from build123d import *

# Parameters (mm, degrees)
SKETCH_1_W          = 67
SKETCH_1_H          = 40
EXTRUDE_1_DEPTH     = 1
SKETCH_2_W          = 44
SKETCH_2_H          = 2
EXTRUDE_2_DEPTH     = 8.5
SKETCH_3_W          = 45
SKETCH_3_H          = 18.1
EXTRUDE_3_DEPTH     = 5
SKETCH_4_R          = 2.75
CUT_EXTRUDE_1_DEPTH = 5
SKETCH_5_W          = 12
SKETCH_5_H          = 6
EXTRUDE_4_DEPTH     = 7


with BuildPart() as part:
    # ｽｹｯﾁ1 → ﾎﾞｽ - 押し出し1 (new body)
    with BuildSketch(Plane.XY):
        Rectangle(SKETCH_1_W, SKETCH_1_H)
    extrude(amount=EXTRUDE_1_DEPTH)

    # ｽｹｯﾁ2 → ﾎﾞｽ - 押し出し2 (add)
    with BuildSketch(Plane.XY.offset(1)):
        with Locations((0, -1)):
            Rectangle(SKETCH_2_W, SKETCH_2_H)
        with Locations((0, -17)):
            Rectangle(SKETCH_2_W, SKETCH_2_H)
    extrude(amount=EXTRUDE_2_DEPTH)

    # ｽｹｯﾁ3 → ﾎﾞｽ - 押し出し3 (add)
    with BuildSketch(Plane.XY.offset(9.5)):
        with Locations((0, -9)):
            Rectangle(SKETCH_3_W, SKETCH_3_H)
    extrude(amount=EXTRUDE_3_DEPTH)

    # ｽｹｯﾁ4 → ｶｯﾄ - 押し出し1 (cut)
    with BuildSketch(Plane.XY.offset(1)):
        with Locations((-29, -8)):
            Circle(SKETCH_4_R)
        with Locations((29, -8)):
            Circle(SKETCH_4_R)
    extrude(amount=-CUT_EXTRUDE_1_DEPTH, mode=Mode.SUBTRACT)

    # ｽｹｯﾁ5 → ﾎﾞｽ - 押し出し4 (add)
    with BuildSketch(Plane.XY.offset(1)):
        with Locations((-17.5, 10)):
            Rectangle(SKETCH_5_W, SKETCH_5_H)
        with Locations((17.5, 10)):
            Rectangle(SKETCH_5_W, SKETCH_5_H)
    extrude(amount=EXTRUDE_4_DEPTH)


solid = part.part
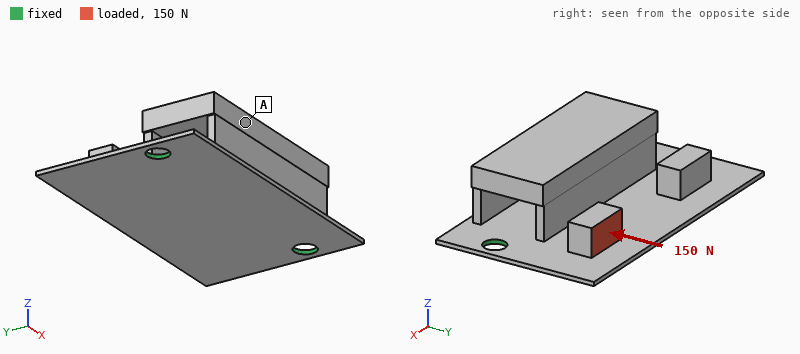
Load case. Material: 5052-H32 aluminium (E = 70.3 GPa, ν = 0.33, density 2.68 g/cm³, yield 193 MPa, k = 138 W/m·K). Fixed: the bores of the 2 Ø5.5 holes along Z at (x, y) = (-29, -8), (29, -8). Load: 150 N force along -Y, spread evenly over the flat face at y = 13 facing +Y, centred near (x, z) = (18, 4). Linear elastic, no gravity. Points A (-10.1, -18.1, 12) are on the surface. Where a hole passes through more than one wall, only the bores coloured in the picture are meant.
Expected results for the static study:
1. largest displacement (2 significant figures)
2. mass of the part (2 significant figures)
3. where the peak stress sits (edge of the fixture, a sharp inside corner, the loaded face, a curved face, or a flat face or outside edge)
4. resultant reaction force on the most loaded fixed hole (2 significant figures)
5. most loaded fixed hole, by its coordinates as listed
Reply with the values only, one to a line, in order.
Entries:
0.49 mm
25 g
a flat face or outside edge
120 N
(29, -8)
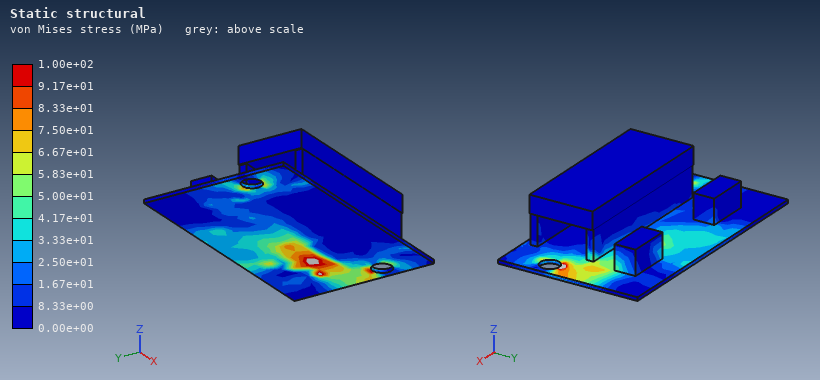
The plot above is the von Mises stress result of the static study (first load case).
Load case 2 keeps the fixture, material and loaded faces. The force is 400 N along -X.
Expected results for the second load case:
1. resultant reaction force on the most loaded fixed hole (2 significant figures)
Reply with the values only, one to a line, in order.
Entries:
250 N
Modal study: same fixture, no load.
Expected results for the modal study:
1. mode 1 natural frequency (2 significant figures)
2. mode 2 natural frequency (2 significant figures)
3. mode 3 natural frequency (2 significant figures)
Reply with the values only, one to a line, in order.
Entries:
820 Hz
1800 Hz
1800 Hz
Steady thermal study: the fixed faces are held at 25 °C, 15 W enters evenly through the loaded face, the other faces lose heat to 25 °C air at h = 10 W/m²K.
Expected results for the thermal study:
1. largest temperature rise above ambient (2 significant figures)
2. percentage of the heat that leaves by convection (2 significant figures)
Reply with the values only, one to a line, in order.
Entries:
64 K
13 %
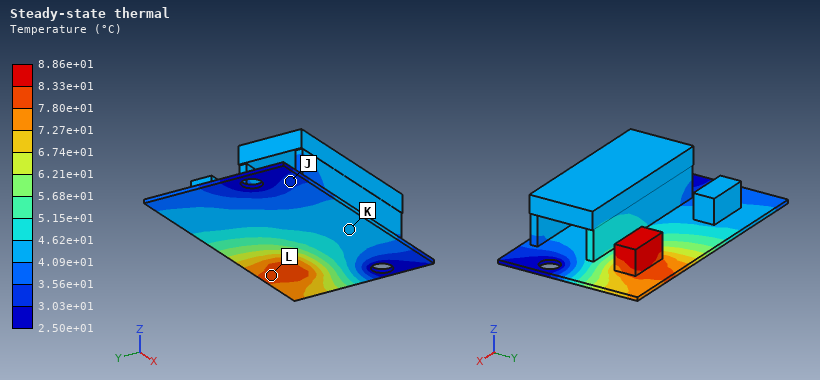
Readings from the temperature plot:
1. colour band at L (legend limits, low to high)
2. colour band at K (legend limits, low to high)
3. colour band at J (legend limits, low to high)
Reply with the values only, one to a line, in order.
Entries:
7.80e+01 to 8.33e+01 °C
4.09e+01 to 4.62e+01 °C
3.03e+01 to 3.56e+01 °C
